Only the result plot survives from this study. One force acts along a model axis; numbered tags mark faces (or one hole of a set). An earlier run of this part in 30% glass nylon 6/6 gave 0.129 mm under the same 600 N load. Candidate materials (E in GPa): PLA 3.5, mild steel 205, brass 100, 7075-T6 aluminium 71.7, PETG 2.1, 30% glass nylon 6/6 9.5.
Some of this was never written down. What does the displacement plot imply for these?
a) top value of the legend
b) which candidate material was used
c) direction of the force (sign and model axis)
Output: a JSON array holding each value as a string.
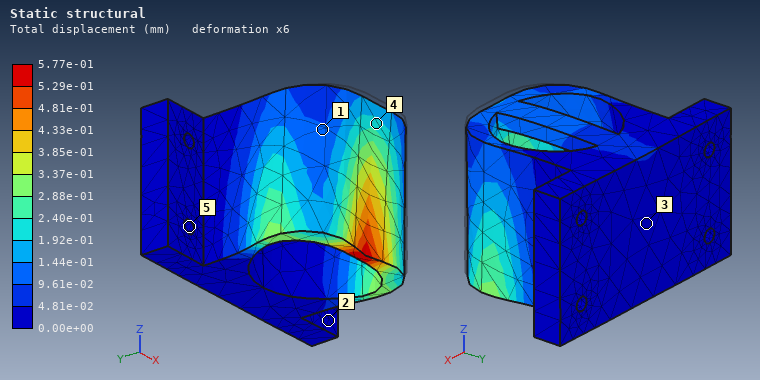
["5.77e-01 mm", "PETG", "+Y"]
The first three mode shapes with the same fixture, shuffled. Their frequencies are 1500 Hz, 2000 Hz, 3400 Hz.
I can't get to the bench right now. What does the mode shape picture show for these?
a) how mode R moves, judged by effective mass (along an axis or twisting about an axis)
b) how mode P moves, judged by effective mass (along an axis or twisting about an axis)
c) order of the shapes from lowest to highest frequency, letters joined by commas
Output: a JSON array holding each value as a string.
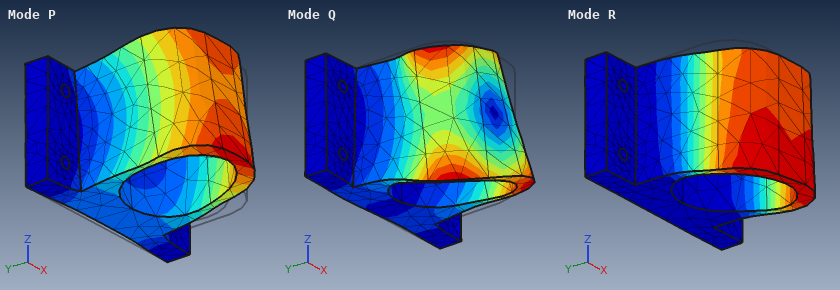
["along X", "along Z", "R, P, Q"]
